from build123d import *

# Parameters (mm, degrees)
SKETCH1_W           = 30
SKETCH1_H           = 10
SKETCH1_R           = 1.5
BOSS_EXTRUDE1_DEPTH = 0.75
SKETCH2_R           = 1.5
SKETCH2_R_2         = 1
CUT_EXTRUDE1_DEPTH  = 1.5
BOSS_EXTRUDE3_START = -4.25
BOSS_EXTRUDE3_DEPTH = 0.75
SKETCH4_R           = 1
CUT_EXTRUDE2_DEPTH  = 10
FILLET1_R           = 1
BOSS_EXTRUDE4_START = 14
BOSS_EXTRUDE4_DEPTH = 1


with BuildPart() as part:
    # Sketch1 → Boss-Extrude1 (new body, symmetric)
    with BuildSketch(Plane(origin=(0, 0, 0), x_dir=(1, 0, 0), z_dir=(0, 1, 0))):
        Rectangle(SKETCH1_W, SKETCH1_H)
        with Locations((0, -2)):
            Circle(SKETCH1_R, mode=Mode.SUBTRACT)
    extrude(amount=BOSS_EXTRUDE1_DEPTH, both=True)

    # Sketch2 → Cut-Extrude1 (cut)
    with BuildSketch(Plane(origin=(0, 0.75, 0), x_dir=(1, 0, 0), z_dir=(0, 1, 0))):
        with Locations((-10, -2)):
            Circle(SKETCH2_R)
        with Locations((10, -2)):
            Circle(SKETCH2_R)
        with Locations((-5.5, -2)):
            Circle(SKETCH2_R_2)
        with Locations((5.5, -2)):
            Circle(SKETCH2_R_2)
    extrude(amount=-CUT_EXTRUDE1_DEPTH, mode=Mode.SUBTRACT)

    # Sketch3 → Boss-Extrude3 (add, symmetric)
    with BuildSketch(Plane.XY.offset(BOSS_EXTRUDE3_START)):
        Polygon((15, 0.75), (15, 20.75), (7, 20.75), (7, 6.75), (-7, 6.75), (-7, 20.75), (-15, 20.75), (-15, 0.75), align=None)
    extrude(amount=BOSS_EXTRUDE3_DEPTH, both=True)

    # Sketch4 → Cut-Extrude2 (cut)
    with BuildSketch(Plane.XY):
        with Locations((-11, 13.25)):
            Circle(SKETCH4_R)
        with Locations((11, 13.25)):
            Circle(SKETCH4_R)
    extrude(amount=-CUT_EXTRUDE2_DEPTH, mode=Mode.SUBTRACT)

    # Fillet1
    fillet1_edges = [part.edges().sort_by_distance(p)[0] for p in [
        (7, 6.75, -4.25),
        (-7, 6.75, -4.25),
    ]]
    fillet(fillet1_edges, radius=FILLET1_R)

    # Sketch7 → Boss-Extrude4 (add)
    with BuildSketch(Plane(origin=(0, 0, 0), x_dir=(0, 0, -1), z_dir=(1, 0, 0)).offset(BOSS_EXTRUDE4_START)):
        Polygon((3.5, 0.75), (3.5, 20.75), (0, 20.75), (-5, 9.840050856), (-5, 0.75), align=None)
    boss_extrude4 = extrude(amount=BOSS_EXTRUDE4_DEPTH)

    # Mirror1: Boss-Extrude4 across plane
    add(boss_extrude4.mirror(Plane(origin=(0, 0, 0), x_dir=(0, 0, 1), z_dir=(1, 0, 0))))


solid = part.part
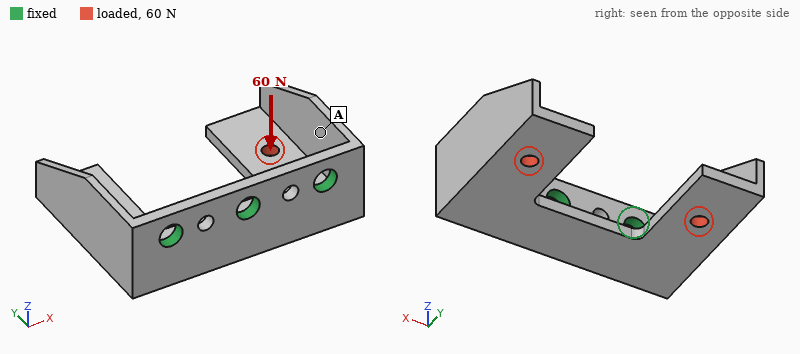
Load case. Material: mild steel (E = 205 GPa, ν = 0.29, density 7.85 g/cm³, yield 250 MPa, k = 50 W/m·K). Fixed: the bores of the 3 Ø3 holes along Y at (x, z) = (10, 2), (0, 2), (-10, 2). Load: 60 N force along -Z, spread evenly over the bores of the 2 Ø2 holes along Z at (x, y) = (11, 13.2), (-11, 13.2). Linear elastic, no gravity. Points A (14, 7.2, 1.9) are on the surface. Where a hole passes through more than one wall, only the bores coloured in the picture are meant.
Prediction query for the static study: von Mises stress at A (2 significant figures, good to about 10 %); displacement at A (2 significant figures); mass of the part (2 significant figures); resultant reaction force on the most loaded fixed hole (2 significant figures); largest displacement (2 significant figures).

12 MPa
7.8 µm
10 g
37 N
29 µm
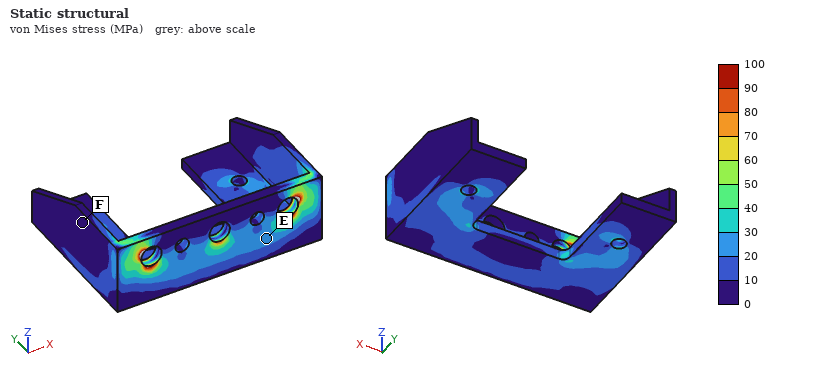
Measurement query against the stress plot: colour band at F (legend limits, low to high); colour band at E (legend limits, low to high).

0 to 10 MPa
20 to 30 MPa
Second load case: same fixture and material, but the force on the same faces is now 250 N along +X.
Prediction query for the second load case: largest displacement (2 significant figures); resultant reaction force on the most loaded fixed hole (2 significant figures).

47 µm
170 N
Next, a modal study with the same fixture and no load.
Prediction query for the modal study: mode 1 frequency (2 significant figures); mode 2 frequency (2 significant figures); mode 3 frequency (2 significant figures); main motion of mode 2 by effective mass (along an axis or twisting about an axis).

4200 Hz
4500 Hz
8800 Hz
along Z
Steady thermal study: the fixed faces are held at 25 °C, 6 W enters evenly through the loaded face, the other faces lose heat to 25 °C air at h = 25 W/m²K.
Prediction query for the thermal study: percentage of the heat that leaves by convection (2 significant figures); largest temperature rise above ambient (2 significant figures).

19 %
50 K
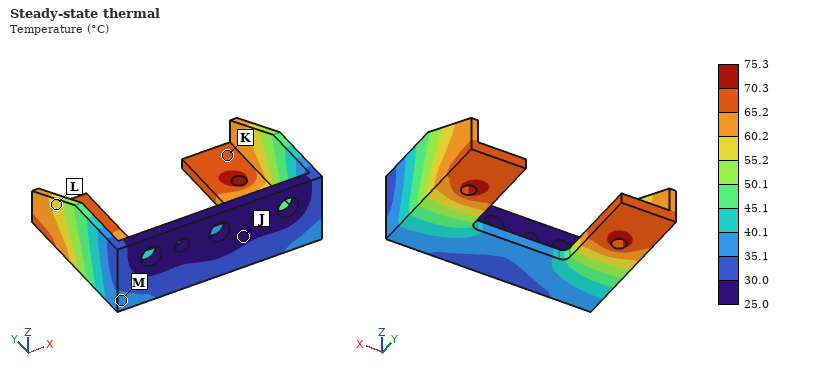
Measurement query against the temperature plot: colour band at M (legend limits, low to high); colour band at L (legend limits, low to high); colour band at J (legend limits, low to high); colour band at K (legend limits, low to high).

35.1 to 40.1 °C
55.2 to 60.2 °C
25.0 to 30.0 °C
65.2 to 70.3 °C
